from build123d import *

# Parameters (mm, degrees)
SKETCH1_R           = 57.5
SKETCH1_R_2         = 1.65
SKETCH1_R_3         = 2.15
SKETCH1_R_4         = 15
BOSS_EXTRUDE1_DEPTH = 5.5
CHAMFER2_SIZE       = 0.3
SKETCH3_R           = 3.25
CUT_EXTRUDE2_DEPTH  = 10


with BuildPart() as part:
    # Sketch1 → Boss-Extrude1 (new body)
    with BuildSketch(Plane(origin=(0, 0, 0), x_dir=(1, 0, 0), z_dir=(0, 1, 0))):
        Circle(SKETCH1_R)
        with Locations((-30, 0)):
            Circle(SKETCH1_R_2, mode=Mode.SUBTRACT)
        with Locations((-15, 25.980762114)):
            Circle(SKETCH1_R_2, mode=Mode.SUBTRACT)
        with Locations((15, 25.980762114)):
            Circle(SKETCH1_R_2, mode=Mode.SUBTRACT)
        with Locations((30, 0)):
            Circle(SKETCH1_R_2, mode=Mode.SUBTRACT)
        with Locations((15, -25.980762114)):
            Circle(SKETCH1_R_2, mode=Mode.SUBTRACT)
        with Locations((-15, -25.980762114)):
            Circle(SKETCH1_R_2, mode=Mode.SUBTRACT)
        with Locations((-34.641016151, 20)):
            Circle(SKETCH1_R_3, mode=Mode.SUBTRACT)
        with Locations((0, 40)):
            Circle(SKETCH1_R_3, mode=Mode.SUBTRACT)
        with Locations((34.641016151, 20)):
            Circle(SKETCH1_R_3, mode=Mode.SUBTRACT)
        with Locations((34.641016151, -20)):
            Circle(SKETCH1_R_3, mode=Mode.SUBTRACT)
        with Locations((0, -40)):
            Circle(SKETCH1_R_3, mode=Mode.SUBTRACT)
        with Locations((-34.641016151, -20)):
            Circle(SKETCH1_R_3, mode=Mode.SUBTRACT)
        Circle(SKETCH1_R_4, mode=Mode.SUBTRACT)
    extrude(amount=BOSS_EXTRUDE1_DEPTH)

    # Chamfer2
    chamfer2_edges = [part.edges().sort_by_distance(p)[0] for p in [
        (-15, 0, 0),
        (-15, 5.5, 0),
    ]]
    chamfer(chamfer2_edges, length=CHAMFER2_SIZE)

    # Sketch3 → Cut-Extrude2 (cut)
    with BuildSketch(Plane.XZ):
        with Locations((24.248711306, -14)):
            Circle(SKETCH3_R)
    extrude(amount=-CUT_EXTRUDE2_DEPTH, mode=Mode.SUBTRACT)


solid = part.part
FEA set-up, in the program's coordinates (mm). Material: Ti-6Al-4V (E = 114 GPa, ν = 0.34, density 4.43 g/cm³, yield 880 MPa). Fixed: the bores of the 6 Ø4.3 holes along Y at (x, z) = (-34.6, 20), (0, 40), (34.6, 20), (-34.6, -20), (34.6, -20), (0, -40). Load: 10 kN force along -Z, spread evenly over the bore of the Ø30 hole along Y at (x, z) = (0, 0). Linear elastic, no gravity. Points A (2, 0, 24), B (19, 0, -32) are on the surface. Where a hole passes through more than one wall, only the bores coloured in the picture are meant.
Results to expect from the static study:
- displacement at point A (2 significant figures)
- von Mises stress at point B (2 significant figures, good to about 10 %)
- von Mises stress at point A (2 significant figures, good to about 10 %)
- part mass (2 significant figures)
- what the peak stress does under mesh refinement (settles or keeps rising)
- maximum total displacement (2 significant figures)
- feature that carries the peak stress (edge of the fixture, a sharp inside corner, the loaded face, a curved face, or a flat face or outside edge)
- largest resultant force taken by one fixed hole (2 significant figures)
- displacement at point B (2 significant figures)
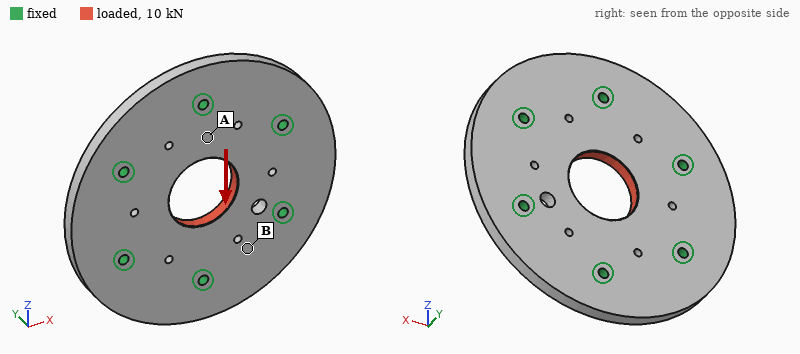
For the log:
3.4 µm
6.1 MPa
22 MPa
230 g
keeps rising
5.6 µm
edge of the fixture
2.4 kN
2.4 µm
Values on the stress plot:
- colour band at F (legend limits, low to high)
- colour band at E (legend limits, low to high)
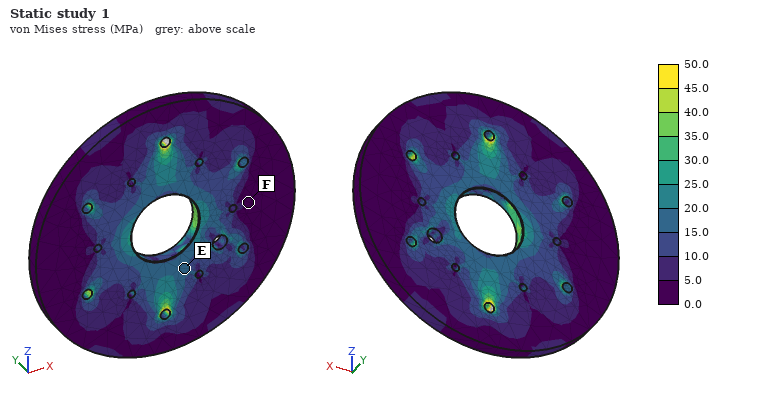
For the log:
0.0 to 5.0 MPa
15.0 to 20.0 MPa
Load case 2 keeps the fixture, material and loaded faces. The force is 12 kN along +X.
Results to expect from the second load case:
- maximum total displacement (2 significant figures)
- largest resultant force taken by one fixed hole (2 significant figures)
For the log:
7.2 µm
2.6 kN
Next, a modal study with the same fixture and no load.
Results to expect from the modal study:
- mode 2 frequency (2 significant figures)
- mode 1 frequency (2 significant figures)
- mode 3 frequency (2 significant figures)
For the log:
7700 Hz
7400 Hz
8100 Hz
